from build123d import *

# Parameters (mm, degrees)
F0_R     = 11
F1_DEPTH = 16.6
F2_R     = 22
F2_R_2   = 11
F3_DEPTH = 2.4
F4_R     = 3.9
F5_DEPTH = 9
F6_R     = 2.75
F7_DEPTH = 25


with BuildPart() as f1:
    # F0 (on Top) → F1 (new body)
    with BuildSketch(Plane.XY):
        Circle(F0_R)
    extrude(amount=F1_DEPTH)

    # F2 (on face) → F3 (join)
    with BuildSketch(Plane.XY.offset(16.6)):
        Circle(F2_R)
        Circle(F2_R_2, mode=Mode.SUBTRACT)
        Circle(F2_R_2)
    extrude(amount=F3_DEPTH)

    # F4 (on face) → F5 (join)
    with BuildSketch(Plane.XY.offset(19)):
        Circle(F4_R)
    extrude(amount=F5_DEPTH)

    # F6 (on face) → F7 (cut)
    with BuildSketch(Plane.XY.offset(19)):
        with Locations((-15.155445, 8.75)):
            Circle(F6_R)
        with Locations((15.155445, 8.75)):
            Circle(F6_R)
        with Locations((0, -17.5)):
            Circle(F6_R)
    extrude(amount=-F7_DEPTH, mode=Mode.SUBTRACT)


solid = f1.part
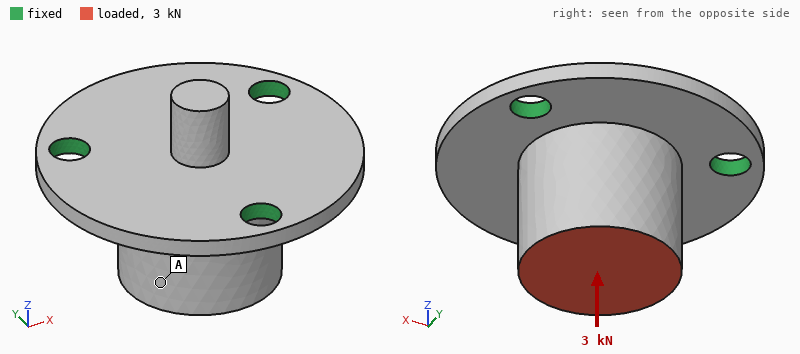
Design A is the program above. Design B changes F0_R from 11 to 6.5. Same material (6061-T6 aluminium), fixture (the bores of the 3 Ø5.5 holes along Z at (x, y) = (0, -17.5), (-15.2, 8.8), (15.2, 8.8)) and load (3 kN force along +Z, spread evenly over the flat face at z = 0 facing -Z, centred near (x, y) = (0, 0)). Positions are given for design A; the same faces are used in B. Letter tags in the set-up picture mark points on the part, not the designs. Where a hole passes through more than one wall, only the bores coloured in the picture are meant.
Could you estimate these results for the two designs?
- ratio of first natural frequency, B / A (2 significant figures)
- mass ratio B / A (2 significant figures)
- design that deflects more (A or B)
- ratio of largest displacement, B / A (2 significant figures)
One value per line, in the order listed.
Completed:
0.86
0.60
B
3.3
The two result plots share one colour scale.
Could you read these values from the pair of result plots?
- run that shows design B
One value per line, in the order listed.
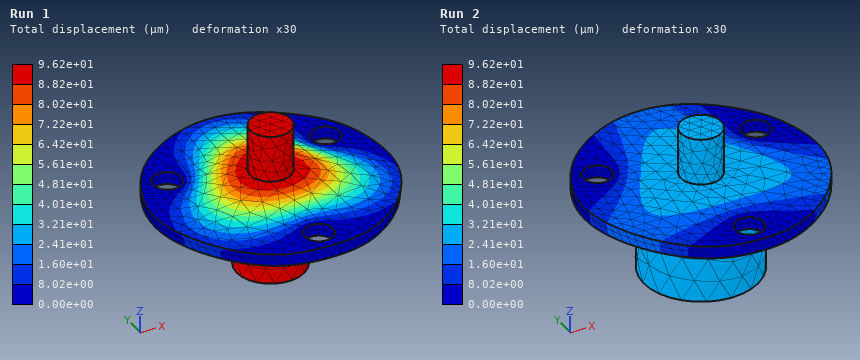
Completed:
Run 1
